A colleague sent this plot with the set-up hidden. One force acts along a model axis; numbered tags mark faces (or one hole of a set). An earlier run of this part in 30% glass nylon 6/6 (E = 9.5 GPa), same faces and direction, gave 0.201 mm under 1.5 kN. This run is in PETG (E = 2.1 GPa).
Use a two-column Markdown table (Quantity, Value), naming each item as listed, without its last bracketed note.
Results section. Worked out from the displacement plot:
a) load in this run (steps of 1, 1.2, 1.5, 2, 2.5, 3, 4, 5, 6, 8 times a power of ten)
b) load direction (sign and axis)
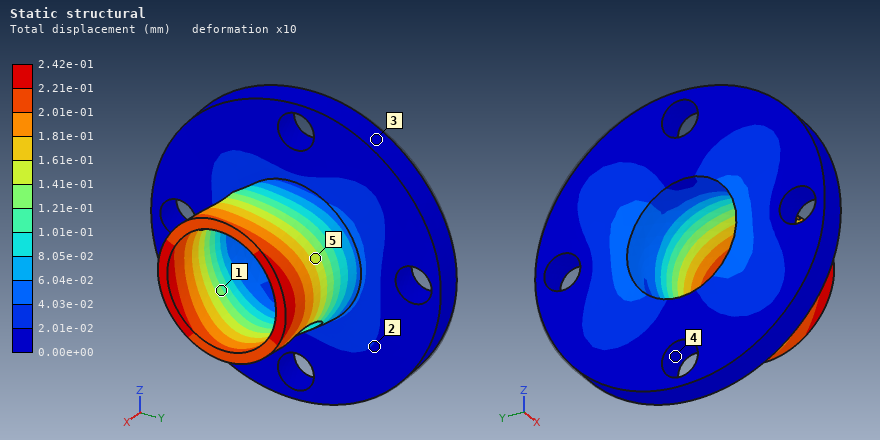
| Quantity | Value |
|---|---|
| load in this run | 400 N |
| load direction | -Y |
